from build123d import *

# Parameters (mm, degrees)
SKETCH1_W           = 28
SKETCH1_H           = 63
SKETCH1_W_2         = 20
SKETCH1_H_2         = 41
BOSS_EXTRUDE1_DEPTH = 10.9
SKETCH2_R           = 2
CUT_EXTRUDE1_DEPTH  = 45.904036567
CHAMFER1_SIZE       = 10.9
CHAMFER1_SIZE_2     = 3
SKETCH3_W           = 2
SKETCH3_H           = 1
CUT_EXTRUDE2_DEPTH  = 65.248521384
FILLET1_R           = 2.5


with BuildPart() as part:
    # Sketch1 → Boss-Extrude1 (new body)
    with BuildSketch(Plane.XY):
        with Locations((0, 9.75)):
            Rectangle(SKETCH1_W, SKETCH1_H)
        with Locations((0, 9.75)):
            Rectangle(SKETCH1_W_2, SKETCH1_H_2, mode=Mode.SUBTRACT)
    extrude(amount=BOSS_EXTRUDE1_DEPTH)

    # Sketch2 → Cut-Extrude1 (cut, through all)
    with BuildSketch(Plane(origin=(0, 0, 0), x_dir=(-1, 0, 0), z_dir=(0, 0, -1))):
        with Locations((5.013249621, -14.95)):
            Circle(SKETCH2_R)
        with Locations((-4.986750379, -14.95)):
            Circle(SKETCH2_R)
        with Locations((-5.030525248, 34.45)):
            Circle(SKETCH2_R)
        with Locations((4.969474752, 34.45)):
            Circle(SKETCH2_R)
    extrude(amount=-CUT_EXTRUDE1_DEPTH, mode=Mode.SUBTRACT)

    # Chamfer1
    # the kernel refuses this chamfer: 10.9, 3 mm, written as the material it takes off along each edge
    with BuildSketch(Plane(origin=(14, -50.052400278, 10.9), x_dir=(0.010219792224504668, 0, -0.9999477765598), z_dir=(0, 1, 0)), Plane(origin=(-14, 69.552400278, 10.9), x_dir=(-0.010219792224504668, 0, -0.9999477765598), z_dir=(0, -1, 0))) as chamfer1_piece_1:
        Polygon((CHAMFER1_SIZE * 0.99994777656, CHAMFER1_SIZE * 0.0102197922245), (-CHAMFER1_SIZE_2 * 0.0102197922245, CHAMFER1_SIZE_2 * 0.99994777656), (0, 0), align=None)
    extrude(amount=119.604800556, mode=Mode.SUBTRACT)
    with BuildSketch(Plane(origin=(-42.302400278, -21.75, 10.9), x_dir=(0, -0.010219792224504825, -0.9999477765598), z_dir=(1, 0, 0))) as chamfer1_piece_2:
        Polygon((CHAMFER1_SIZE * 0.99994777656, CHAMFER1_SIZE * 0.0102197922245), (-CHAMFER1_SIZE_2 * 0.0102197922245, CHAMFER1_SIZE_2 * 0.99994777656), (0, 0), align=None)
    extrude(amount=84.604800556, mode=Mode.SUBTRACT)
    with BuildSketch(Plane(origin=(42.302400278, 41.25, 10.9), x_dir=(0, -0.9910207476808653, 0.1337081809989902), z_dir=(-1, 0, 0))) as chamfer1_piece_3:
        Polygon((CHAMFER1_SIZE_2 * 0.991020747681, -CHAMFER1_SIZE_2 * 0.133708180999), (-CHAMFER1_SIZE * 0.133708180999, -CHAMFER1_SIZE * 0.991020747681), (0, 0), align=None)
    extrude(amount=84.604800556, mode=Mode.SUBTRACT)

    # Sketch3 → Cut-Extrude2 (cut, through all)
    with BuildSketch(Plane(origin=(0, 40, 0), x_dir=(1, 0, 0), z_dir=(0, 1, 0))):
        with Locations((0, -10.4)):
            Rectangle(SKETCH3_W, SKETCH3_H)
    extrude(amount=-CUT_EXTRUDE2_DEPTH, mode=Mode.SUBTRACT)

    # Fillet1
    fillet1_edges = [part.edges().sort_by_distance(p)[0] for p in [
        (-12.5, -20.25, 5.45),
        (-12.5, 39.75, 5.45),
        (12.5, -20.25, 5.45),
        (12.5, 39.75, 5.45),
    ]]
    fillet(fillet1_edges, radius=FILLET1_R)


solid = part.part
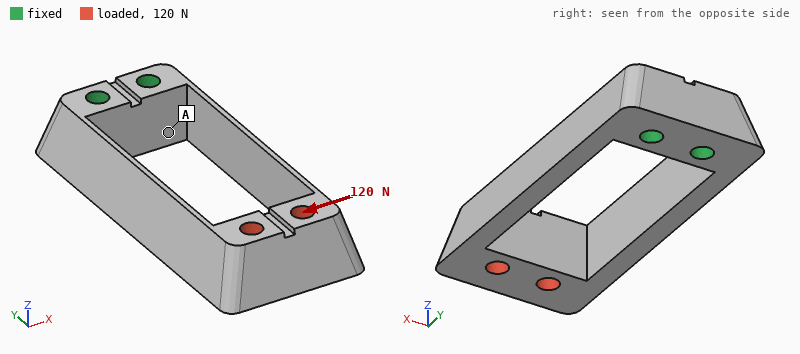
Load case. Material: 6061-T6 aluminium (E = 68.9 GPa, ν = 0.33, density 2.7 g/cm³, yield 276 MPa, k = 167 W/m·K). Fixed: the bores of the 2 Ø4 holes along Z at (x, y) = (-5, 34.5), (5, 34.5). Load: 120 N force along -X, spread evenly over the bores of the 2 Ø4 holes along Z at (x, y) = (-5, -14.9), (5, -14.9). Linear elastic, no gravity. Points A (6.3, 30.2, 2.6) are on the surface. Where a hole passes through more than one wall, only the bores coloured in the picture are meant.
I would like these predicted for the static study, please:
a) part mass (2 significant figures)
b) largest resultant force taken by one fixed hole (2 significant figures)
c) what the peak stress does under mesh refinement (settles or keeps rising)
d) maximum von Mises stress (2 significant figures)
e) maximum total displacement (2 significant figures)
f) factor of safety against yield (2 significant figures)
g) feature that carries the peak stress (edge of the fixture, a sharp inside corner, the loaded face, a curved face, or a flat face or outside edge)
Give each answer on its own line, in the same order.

18 g
270 N
settles
120 MPa
0.35 mm
2.3
a flat face or outside edge
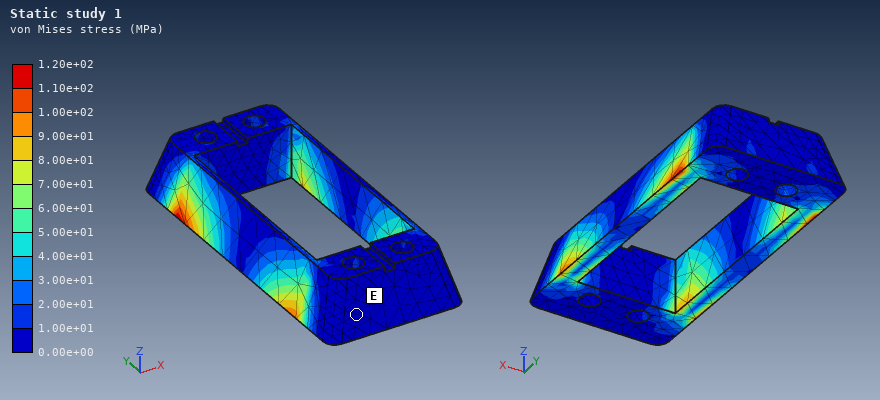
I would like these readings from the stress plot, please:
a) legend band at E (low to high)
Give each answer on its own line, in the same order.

0.00e+00 to 1.00e+01 MPa
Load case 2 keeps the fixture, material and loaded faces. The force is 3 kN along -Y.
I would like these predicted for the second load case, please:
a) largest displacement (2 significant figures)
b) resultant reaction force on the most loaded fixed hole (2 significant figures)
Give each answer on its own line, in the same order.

0.15 mm
1.5 kN
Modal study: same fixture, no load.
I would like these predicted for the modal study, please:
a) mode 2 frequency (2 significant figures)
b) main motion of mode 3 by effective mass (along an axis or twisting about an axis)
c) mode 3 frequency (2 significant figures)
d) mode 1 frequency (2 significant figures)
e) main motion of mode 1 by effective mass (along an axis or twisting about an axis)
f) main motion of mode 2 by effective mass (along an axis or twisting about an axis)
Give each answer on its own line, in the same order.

1600 Hz
twisting about Y
3700 Hz
1000 Hz
along X
along Z
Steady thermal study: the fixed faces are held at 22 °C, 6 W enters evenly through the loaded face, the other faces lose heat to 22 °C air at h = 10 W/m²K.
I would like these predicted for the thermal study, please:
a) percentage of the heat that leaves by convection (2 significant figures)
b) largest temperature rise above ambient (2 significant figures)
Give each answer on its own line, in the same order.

11 %
29 K
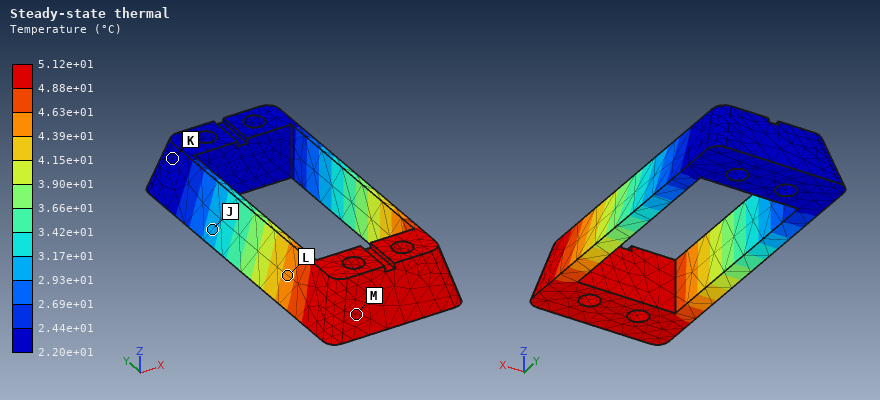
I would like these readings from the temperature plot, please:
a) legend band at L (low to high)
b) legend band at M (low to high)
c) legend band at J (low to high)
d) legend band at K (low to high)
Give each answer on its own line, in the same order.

4.39e+01 to 4.63e+01 °C
4.88e+01 to 5.12e+01 °C
2.93e+01 to 3.17e+01 °C
2.20e+01 to 2.44e+01 °C
